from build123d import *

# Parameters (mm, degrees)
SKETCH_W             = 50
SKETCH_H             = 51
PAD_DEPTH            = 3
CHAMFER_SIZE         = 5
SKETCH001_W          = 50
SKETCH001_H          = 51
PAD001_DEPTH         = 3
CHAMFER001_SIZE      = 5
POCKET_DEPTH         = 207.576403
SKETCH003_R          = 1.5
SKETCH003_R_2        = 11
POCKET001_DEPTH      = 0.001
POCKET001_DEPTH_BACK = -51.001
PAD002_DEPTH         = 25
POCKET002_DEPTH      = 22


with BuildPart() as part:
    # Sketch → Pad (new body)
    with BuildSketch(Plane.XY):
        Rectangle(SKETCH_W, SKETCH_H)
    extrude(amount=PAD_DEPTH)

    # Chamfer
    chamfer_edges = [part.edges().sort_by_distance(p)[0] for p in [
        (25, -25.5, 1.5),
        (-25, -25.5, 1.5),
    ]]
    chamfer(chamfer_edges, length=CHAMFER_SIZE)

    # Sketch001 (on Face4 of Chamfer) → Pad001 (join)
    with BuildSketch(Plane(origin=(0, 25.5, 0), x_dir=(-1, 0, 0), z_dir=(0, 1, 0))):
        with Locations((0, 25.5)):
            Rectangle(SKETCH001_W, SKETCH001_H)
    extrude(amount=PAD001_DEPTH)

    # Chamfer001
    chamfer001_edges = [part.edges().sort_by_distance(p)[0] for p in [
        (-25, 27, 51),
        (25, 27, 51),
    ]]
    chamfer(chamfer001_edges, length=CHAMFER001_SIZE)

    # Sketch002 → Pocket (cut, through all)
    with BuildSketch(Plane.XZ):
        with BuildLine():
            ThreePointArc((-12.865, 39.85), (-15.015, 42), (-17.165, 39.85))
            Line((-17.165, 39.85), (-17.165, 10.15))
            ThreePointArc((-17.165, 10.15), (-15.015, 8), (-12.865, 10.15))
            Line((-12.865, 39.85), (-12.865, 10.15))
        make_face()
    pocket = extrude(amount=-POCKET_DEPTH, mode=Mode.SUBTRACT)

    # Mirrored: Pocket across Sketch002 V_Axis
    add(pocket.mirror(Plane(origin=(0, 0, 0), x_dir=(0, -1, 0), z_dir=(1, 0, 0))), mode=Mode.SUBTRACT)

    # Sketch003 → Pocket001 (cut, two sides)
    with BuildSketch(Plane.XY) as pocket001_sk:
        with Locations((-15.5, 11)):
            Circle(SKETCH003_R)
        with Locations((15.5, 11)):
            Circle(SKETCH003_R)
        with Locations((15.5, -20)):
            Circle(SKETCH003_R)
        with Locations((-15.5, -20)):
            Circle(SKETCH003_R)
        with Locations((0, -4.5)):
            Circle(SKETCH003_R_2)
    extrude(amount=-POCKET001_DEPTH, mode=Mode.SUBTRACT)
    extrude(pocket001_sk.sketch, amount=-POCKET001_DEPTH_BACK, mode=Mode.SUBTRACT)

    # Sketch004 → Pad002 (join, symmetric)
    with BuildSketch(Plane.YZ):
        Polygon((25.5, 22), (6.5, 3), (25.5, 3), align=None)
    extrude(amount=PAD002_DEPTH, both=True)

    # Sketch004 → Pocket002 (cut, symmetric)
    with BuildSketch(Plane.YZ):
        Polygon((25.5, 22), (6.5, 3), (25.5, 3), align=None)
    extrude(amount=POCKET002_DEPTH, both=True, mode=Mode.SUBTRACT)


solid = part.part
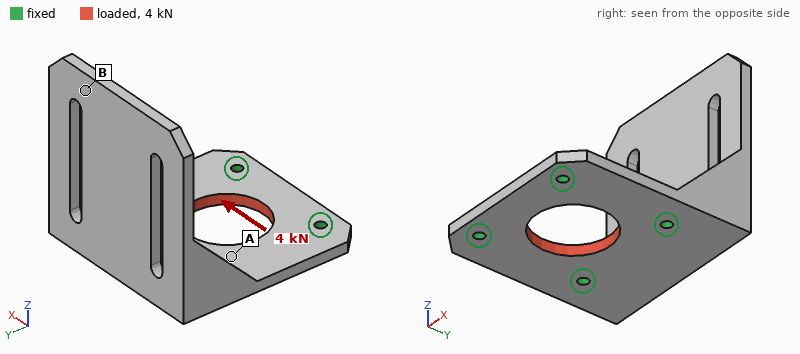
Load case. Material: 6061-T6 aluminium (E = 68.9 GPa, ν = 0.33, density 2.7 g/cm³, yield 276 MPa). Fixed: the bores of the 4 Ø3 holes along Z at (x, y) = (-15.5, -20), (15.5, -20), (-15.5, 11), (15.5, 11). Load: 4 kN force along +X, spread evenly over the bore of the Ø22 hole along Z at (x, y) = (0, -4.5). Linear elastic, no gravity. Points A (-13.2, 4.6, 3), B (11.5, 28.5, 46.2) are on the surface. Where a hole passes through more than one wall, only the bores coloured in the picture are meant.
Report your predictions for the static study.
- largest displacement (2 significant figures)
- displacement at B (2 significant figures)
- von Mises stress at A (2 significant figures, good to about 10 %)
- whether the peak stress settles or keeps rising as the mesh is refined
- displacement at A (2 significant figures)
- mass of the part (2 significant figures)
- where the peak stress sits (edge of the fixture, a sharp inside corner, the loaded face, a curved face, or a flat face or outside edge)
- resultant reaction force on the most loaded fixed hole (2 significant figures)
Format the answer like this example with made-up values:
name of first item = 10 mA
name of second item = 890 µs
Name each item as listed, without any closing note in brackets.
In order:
largest displacement = 9.6 µm
displacement at B = 1.9 µm
von Mises stress at A = 23 MPa
whether the peak stress settles or keeps rising as the mesh is refined = keeps rising
displacement at A = 4.9 µm
mass of the part = 38 g
where the peak stress sits = edge of the fixture
resultant reaction force on the most loaded fixed hole = 1.0 kN
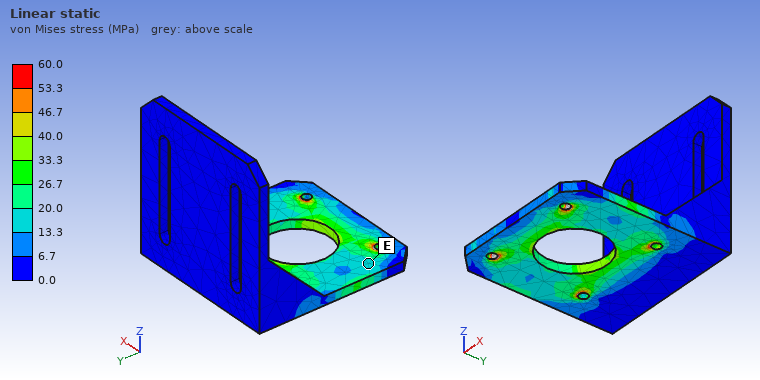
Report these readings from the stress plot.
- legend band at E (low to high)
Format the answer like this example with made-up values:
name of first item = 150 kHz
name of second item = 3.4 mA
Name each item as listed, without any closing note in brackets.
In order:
legend band at E = 13.3 to 20.0 MPa
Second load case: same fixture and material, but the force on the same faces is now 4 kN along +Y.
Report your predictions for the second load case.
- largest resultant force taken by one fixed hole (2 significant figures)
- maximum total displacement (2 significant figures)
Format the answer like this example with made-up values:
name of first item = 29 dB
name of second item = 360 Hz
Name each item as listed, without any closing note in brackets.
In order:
largest resultant force taken by one fixed hole = 1.0 kN
maximum total displacement = 13 µm
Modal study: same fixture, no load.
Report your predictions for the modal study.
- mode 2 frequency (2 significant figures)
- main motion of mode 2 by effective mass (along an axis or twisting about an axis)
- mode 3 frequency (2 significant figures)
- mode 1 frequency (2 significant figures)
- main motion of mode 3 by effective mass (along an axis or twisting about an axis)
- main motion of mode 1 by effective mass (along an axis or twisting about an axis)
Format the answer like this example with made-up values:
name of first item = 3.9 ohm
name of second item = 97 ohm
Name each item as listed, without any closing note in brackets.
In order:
mode 2 frequency = 1900 Hz
main motion of mode 2 by effective mass = along X
mode 3 frequency = 3500 Hz
mode 1 frequency = 1100 Hz
main motion of mode 3 by effective mass = along Z
main motion of mode 1 by effective mass = along Y
